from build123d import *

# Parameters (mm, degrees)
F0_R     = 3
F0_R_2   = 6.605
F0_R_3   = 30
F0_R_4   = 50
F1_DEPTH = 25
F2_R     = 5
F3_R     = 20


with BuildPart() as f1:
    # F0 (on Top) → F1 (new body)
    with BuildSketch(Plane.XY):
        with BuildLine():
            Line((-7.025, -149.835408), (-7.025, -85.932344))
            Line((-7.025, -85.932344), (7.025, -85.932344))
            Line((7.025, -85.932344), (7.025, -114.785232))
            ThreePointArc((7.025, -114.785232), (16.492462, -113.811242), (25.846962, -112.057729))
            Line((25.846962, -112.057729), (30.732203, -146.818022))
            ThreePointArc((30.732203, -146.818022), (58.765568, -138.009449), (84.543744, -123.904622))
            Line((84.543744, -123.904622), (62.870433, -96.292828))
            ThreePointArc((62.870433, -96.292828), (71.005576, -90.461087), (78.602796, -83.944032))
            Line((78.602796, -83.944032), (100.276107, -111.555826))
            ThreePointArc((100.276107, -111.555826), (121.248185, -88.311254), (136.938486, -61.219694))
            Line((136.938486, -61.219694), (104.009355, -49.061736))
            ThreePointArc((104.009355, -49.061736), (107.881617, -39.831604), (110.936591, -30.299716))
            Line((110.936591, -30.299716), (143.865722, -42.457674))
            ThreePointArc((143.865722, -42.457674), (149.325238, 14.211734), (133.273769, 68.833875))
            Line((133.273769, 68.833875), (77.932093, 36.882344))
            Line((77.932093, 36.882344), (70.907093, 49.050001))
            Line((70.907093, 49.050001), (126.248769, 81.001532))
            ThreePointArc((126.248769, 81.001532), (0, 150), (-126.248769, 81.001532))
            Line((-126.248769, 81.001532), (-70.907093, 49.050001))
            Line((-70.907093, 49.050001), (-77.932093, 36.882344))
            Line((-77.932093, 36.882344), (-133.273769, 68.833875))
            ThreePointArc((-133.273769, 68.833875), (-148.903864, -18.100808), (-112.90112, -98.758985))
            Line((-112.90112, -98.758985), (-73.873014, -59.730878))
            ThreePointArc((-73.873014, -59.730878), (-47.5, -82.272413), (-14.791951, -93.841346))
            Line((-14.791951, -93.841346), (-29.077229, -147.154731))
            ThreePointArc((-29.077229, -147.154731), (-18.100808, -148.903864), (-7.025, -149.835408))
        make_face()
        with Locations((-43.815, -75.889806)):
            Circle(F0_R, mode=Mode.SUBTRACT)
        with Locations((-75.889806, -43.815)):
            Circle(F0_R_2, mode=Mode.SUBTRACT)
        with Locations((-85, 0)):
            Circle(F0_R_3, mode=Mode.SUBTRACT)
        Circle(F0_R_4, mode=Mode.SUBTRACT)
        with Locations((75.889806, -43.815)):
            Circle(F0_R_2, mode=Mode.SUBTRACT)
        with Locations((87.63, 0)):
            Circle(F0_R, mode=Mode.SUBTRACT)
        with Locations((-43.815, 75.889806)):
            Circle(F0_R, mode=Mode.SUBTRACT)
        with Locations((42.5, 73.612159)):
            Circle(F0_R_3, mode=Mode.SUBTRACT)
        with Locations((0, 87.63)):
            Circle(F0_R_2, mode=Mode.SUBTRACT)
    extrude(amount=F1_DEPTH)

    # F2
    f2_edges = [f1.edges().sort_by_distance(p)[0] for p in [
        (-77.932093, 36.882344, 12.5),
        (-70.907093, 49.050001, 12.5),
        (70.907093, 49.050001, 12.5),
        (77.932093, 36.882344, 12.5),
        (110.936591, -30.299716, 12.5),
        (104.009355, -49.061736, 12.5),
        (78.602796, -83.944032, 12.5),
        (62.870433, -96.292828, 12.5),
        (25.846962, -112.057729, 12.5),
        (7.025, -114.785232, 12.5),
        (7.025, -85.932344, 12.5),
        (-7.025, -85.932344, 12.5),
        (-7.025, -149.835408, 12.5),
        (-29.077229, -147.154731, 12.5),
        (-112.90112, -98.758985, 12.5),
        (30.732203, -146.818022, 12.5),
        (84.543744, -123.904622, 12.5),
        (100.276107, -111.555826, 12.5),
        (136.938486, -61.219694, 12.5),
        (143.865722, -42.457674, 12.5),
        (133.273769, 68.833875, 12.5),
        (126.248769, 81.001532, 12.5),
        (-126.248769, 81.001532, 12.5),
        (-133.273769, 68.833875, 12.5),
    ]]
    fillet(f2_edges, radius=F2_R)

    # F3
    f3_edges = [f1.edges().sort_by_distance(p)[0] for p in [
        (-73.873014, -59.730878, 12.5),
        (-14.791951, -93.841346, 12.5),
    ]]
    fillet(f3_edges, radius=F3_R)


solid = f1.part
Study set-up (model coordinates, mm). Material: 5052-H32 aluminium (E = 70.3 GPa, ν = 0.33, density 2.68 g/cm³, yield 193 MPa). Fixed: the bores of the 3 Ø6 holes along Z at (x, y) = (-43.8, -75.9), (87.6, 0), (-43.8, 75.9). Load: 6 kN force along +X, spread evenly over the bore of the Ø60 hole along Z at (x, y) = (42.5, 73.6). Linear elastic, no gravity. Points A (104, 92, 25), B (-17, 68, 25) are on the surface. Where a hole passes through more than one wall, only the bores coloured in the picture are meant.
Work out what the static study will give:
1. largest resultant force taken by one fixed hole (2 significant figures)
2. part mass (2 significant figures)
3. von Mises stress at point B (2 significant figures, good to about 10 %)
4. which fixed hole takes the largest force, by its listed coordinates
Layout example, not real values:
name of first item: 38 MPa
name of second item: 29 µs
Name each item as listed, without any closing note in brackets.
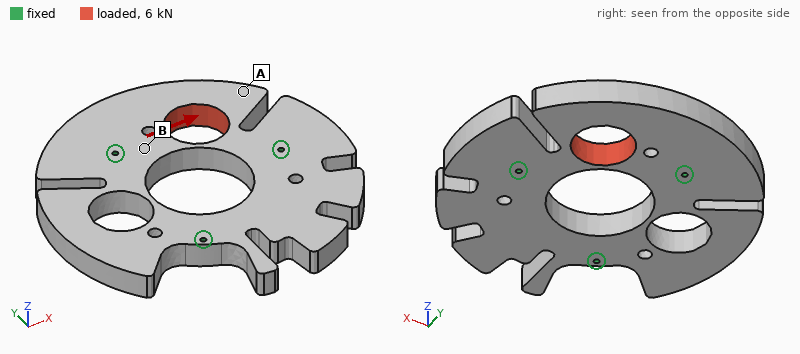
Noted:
largest resultant force taken by one fixed hole: 4.1 kN
part mass: 3.2 kg
von Mises stress at point B: 2.9 MPa
which fixed hole takes the largest force, by its listed coordinates: (-43.8, 75.9)
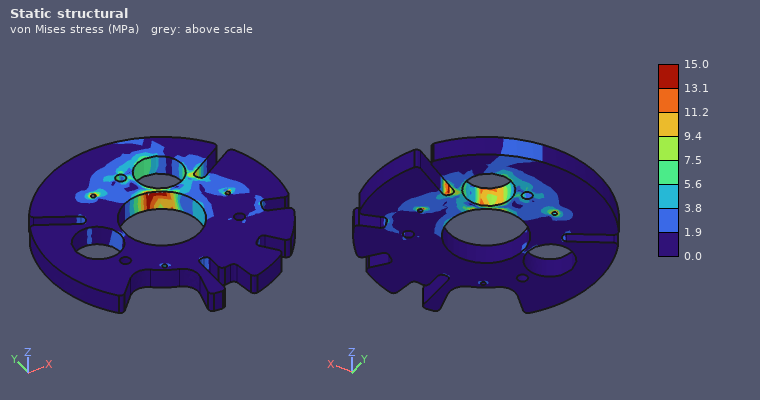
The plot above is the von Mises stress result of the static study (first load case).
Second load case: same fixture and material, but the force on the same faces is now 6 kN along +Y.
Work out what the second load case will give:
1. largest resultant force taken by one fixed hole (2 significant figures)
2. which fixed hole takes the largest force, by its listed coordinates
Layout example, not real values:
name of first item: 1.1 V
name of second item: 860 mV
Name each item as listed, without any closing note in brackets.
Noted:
largest resultant force taken by one fixed hole: 4.3 kN
which fixed hole takes the largest force, by its listed coordinates: (87.6, 0)
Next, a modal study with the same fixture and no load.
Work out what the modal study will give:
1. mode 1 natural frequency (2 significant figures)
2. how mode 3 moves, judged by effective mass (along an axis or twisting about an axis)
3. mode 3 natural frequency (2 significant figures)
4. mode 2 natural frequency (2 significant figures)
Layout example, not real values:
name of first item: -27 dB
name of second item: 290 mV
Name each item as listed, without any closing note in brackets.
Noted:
mode 1 natural frequency: 1100 Hz
how mode 3 moves, judged by effective mass: along Z
mode 3 natural frequency: 1400 Hz
mode 2 natural frequency: 1200 Hz
